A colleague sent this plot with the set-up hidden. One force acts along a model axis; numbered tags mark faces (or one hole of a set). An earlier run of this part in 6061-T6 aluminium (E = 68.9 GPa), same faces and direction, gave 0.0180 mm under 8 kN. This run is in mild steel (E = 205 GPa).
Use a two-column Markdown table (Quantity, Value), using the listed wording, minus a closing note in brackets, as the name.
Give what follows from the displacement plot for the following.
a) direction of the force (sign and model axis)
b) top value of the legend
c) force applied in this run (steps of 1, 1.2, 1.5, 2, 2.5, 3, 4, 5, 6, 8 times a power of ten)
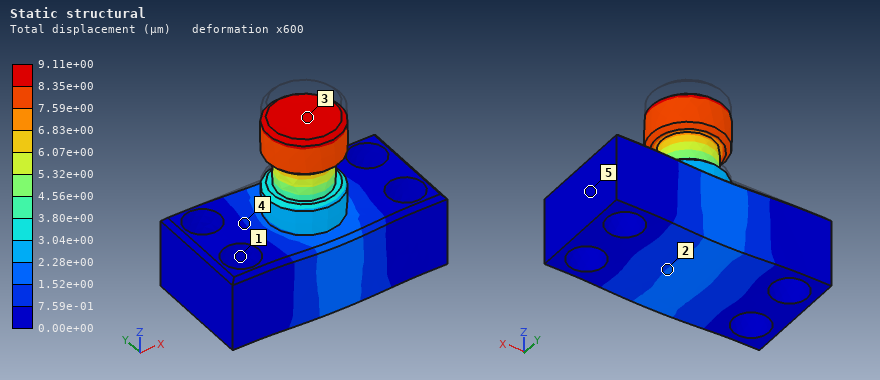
| Quantity | Value |
|---|---|
| direction of the force | -Z |
| top value of the legend | 9.11e+00 µm |
| force applied in this run | 12 kN |
